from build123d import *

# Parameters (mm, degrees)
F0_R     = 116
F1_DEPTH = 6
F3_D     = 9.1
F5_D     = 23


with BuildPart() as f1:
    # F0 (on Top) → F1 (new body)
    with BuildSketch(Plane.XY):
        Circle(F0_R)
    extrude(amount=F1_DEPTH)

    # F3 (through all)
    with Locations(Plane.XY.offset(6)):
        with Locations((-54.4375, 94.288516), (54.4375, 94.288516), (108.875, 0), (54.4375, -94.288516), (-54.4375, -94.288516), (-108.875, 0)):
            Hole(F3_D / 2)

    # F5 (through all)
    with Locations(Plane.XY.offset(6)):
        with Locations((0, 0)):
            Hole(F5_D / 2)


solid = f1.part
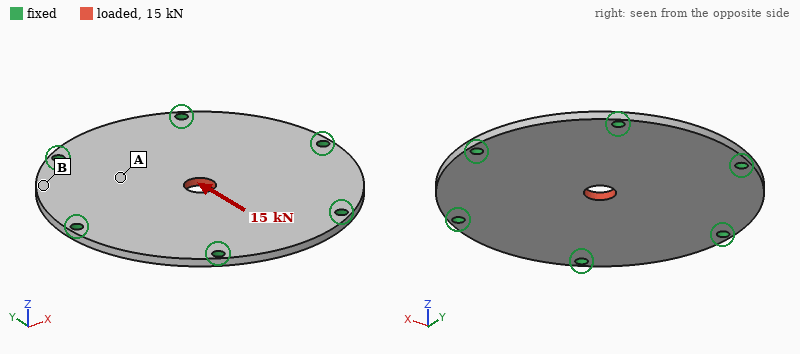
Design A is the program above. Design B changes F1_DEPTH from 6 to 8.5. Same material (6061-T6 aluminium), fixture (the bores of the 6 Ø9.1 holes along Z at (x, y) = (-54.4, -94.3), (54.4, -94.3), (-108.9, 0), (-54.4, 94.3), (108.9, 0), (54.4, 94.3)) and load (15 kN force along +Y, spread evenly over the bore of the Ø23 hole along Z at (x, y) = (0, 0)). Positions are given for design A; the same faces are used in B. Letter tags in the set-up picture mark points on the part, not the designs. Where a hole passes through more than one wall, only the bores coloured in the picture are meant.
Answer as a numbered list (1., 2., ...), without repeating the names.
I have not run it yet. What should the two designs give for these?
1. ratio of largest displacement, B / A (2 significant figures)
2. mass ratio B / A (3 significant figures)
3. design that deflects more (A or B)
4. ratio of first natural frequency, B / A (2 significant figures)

1. 0.71
2. 1.42
3. A
4. 1.4
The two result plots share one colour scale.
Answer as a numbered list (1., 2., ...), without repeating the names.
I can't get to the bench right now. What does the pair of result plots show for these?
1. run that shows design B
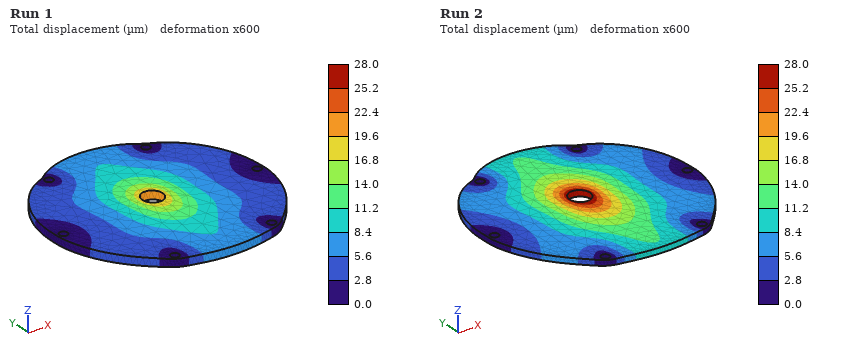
1. Run 1
